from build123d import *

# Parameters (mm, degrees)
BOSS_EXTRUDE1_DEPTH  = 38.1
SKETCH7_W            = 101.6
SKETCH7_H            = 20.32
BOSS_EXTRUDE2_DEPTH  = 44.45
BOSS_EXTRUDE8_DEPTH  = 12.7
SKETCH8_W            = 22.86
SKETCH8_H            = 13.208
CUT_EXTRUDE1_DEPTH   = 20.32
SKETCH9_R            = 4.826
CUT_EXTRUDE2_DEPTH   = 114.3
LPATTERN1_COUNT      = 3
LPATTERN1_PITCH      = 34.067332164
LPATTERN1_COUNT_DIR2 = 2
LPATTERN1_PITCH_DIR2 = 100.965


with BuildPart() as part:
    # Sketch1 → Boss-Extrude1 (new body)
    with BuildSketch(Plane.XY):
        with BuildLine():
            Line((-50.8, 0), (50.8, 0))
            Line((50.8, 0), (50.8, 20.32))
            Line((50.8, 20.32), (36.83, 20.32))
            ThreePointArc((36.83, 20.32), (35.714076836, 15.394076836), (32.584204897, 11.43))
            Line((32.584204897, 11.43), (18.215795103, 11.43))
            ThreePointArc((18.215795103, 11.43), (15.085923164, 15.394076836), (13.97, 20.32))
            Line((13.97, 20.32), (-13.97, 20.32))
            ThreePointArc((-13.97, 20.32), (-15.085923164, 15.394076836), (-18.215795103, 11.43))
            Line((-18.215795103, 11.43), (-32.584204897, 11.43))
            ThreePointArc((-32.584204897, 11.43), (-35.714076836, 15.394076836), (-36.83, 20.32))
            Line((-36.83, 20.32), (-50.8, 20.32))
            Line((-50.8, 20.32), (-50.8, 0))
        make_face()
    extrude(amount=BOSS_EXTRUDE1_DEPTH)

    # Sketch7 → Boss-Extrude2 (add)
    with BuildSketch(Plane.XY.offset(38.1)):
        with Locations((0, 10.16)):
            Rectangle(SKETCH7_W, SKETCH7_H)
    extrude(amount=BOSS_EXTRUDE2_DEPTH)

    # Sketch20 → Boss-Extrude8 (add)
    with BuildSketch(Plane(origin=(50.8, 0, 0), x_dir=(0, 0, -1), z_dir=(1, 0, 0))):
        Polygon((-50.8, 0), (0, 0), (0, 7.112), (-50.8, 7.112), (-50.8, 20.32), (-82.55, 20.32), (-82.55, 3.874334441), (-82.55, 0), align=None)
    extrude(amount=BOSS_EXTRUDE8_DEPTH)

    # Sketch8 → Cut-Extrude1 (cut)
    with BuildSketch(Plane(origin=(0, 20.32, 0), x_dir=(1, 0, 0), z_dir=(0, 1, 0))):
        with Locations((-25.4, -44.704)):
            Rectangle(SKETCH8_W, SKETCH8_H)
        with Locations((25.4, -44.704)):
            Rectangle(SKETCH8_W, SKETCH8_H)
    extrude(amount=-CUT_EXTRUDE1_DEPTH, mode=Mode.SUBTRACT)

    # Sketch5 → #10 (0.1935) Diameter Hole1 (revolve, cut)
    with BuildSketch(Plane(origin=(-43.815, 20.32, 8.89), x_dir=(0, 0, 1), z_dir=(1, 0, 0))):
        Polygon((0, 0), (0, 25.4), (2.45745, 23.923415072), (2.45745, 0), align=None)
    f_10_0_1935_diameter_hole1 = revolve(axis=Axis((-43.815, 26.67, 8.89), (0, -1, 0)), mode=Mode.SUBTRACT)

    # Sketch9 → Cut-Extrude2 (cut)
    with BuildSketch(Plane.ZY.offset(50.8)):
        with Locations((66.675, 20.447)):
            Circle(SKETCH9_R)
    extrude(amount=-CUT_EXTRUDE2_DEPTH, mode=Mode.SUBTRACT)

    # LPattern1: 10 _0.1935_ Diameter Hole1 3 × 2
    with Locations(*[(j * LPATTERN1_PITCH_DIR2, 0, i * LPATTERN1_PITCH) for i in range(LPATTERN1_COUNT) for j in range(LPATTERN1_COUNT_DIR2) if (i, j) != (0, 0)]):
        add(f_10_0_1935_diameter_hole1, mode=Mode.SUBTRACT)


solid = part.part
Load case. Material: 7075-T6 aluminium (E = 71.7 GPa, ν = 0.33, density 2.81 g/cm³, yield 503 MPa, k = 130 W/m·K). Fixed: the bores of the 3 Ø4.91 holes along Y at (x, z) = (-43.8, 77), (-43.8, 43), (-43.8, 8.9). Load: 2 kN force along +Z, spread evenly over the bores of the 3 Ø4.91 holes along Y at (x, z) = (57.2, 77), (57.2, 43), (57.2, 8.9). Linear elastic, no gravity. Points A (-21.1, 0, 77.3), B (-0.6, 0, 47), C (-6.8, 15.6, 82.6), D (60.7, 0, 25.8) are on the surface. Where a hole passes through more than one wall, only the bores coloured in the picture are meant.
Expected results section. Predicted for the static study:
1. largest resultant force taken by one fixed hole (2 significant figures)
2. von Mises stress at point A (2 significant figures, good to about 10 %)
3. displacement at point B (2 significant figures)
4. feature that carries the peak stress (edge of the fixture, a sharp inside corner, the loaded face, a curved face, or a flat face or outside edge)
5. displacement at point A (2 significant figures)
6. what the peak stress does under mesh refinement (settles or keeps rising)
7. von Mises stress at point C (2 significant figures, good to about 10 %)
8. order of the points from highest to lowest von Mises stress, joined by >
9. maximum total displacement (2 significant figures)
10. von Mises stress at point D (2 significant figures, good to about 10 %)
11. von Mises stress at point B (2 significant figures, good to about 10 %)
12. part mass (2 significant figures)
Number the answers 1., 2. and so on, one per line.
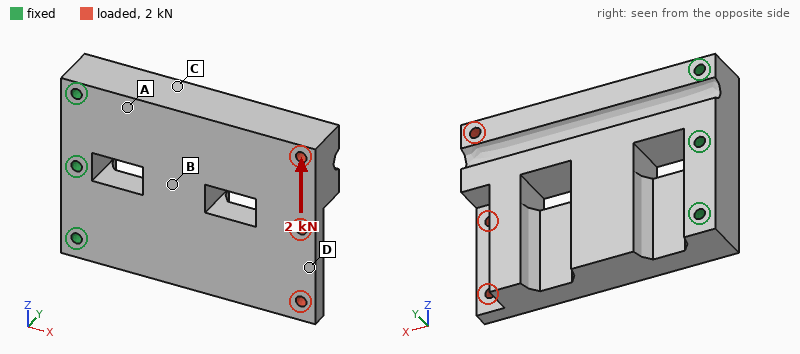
1. 3.0 kN
2. 10 MPa
3. 9.9 µm
4. edge of the fixture
5. 5.9 µm
6. keeps rising
7. 5.4 MPa
8. A > B > C > D
9. 39 µm
10. 2.2 MPa
11. 8.6 MPa
12. 430 g
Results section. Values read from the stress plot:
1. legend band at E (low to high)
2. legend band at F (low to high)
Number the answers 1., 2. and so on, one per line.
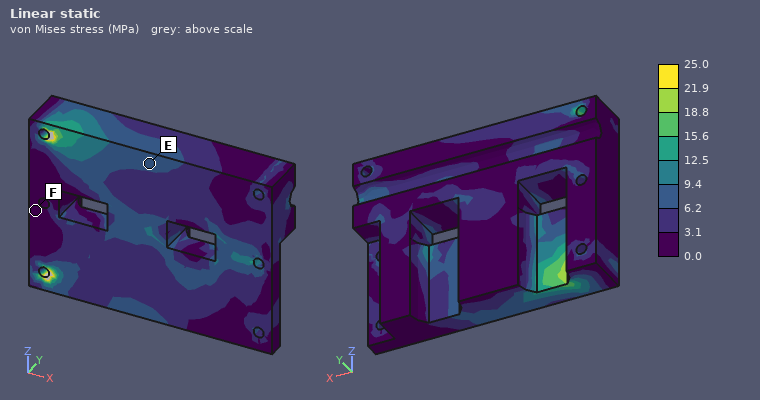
1. 6.2 to 9.4 MPa
2. 0.0 to 3.1 MPa
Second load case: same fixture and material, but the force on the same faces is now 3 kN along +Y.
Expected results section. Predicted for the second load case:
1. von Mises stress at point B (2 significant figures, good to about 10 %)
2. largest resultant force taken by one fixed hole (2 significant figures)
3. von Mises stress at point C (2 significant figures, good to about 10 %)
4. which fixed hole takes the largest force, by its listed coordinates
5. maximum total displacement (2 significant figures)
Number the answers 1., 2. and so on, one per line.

1. 23 MPa
2. 1.9 kN
3. 39 MPa
4. (-43.8, 77)
5. 0.66 mm
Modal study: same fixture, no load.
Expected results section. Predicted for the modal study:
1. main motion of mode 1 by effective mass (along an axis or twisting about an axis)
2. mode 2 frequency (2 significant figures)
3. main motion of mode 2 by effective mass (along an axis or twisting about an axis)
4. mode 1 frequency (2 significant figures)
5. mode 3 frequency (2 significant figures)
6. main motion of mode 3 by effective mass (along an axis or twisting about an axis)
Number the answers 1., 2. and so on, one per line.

1. along Y
2. 3000 Hz
3. twisting about X
4. 1100 Hz
5. 3900 Hz
6. along Z
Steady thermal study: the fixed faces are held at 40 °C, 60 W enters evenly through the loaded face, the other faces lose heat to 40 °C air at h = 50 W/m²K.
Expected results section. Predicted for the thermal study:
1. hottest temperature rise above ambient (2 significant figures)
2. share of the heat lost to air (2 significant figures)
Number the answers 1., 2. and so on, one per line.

1. 40 K
2. 35 %
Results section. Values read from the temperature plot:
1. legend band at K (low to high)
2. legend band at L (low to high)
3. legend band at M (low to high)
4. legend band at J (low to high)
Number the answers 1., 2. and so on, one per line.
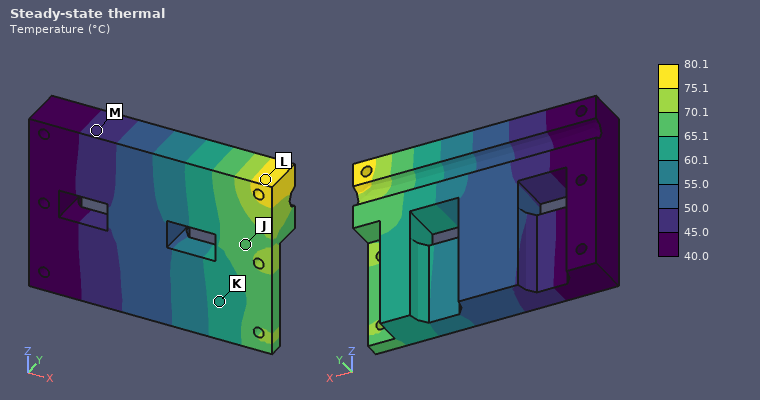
1. 60.1 to 65.1 °C
2. 75.1 to 80.1 °C
3. 45.0 to 50.0 °C
4. 65.1 to 70.1 °C
